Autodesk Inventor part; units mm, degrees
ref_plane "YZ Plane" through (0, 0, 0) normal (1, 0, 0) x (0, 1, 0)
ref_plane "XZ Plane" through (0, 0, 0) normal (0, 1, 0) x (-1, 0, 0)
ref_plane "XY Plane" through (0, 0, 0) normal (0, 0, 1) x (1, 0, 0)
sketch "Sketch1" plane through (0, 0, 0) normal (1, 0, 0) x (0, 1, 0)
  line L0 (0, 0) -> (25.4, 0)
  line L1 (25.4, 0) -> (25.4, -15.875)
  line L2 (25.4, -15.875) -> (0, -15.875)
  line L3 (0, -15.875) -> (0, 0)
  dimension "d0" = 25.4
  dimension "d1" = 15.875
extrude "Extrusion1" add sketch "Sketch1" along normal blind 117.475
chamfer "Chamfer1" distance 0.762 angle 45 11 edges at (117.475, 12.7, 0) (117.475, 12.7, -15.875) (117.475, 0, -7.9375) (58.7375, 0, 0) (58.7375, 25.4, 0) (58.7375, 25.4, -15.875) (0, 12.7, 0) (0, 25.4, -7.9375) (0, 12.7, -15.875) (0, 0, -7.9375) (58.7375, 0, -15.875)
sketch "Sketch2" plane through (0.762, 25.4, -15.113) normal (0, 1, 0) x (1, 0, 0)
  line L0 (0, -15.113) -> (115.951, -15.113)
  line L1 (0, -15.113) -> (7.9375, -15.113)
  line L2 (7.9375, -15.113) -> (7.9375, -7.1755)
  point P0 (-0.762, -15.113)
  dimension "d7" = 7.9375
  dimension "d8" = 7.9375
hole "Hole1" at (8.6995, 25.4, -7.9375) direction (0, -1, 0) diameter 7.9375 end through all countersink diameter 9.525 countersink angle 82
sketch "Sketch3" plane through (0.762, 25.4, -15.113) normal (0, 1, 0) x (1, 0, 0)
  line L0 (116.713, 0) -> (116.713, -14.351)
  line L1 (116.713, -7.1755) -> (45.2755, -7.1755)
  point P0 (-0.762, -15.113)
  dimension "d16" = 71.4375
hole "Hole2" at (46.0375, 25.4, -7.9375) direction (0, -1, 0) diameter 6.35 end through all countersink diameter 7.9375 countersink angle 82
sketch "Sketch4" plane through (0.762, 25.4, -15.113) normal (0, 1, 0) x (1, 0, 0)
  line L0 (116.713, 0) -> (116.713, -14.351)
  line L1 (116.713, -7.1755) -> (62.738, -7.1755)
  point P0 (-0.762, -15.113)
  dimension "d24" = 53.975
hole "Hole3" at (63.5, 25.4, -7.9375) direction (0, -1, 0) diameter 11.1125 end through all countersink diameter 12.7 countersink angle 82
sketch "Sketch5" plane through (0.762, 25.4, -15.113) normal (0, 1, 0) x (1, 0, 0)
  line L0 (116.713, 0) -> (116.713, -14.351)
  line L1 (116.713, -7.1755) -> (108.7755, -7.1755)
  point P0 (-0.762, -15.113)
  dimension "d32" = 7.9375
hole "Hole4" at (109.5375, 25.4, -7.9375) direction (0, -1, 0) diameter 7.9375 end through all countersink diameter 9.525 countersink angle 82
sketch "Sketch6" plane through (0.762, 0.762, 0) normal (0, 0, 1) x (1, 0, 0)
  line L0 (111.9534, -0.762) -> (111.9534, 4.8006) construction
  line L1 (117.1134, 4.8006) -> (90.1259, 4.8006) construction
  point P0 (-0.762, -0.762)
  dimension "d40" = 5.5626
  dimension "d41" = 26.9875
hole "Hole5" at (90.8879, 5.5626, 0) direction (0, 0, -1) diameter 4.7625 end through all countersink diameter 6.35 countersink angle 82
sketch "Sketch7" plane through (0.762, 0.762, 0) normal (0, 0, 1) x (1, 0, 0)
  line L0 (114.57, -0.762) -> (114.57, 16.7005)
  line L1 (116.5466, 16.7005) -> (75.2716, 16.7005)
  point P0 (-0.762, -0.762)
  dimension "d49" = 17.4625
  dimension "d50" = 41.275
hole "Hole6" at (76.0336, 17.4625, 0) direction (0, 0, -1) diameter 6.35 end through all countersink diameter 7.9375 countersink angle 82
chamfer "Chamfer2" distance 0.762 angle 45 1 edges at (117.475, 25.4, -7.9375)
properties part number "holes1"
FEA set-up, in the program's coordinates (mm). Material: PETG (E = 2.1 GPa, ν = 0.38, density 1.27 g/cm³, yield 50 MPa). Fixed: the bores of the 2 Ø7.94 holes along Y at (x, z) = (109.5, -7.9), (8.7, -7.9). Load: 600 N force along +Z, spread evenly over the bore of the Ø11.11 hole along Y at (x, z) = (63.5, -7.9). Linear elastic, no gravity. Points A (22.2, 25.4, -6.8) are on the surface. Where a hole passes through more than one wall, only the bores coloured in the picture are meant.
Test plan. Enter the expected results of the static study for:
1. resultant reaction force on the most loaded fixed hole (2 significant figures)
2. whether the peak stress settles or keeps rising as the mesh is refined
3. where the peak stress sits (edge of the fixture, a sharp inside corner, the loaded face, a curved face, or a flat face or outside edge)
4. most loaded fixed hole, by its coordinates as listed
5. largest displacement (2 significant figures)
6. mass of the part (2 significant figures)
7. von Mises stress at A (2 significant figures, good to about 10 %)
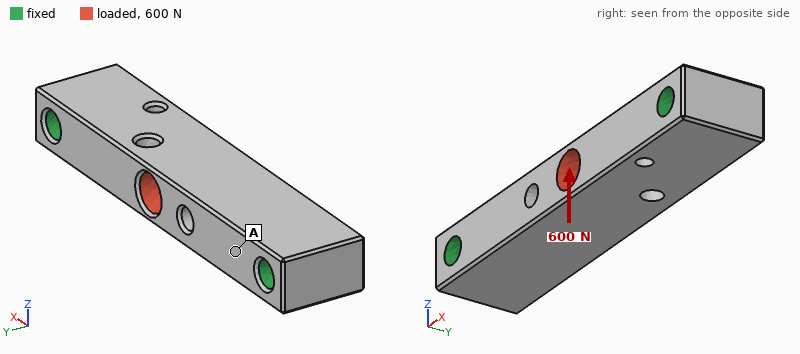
340 N
keeps rising
edge of the fixture
(109.5, -7.9)
0.28 mm
52 g
1.8 MPa
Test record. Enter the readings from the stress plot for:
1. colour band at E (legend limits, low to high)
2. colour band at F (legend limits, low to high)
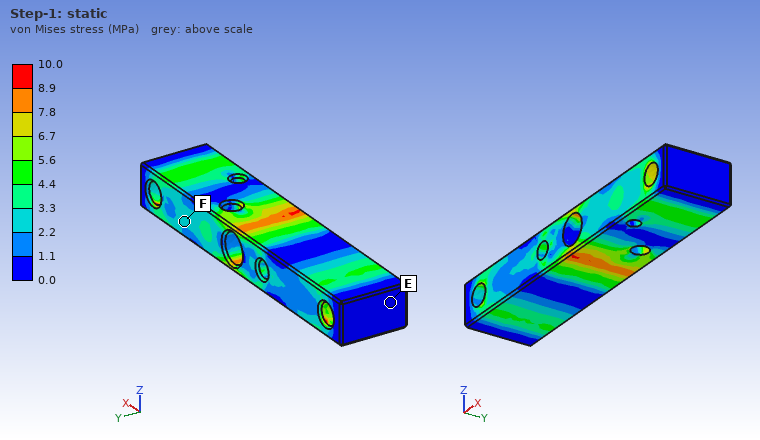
0.0 to 1.1 MPa
2.2 to 3.3 MPa
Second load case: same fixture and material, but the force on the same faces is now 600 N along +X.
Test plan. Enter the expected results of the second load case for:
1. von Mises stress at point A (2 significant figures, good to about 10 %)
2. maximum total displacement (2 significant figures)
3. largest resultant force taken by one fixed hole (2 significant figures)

0.73 MPa
20 µm
320 N
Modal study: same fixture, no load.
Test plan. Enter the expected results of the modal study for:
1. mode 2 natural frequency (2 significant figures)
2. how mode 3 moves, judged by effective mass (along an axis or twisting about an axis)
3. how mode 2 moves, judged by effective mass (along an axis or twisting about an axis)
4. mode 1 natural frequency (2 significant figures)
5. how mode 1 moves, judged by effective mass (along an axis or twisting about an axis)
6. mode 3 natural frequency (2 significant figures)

2600 Hz
twisting about X
along Y
1900 Hz
along Z
3600 Hz
